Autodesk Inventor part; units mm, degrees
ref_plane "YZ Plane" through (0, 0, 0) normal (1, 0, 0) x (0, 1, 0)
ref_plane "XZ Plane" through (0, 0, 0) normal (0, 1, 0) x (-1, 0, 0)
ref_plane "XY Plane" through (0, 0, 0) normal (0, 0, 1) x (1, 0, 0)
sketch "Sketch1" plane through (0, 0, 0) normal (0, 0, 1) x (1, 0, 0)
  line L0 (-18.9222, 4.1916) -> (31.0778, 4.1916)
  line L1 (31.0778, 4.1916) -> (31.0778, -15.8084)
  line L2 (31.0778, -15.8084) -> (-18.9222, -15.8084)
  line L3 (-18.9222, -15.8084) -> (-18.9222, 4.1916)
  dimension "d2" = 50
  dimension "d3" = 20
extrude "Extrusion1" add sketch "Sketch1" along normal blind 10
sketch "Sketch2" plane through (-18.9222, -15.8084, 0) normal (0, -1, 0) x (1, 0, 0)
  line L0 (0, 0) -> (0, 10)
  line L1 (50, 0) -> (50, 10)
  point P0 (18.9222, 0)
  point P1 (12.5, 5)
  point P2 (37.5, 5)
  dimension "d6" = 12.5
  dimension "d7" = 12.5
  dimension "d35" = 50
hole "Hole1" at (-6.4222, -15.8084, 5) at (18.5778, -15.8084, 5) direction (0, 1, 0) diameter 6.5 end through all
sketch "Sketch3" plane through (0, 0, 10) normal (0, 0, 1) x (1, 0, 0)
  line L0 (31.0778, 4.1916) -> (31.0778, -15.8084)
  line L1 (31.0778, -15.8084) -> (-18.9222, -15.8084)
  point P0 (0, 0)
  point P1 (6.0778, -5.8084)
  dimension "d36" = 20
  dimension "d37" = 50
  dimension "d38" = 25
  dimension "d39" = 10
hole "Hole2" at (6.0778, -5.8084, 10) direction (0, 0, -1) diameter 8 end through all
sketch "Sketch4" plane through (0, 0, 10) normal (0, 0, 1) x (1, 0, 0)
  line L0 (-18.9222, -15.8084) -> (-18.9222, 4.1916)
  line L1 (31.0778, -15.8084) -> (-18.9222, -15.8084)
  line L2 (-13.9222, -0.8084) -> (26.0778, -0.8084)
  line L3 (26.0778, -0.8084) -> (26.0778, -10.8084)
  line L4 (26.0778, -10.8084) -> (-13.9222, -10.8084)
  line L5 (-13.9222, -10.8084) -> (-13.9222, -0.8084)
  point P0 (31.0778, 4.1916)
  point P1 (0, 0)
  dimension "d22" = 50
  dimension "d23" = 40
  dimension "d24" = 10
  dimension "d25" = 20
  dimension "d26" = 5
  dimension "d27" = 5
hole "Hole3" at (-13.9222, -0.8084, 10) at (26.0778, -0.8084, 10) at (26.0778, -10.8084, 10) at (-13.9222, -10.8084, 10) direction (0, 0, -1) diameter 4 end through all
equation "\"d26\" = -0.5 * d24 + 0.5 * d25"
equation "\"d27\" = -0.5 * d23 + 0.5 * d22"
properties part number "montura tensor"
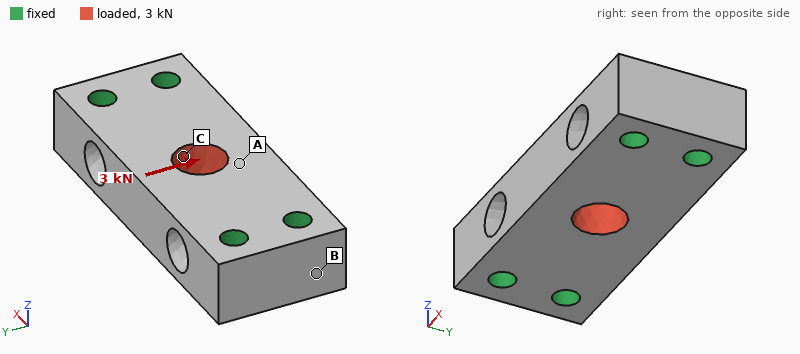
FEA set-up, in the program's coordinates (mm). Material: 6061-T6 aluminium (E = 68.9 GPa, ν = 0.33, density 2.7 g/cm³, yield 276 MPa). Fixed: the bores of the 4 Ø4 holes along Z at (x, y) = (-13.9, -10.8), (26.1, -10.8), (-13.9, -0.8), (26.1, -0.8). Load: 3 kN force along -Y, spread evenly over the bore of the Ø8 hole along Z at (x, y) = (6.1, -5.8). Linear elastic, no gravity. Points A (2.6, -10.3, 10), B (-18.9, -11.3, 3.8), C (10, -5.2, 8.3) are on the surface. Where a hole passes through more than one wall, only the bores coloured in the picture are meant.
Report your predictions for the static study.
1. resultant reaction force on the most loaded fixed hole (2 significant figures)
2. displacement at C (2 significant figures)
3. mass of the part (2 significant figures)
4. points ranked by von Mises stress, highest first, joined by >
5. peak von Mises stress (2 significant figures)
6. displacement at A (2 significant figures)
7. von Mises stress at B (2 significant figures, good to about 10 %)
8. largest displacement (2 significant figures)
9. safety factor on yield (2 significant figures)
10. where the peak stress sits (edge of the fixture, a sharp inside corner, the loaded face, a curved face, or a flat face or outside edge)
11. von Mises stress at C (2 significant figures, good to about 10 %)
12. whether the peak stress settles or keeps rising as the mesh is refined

1.1 kN
11 µm
21 g
C > A > B
61 MPa
11 µm
4.9 MPa
12 µm
4.6
a curved face
23 MPa
settles
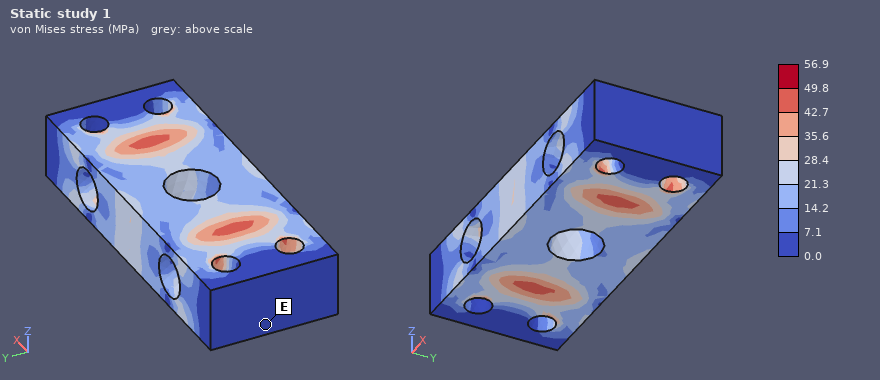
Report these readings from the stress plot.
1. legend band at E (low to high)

0.0 to 7.1 MPa
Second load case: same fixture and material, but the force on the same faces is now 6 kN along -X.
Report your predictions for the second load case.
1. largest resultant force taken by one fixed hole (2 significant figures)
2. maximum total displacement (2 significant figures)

1.5 kN
8.4 µm
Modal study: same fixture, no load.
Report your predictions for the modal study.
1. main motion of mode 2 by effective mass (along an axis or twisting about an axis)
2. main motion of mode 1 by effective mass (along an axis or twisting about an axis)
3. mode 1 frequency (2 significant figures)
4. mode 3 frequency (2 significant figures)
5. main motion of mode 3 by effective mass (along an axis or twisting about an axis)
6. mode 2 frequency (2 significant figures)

twisting about X
along Z
17 kHz
28 kHz
along Y
25 kHz
